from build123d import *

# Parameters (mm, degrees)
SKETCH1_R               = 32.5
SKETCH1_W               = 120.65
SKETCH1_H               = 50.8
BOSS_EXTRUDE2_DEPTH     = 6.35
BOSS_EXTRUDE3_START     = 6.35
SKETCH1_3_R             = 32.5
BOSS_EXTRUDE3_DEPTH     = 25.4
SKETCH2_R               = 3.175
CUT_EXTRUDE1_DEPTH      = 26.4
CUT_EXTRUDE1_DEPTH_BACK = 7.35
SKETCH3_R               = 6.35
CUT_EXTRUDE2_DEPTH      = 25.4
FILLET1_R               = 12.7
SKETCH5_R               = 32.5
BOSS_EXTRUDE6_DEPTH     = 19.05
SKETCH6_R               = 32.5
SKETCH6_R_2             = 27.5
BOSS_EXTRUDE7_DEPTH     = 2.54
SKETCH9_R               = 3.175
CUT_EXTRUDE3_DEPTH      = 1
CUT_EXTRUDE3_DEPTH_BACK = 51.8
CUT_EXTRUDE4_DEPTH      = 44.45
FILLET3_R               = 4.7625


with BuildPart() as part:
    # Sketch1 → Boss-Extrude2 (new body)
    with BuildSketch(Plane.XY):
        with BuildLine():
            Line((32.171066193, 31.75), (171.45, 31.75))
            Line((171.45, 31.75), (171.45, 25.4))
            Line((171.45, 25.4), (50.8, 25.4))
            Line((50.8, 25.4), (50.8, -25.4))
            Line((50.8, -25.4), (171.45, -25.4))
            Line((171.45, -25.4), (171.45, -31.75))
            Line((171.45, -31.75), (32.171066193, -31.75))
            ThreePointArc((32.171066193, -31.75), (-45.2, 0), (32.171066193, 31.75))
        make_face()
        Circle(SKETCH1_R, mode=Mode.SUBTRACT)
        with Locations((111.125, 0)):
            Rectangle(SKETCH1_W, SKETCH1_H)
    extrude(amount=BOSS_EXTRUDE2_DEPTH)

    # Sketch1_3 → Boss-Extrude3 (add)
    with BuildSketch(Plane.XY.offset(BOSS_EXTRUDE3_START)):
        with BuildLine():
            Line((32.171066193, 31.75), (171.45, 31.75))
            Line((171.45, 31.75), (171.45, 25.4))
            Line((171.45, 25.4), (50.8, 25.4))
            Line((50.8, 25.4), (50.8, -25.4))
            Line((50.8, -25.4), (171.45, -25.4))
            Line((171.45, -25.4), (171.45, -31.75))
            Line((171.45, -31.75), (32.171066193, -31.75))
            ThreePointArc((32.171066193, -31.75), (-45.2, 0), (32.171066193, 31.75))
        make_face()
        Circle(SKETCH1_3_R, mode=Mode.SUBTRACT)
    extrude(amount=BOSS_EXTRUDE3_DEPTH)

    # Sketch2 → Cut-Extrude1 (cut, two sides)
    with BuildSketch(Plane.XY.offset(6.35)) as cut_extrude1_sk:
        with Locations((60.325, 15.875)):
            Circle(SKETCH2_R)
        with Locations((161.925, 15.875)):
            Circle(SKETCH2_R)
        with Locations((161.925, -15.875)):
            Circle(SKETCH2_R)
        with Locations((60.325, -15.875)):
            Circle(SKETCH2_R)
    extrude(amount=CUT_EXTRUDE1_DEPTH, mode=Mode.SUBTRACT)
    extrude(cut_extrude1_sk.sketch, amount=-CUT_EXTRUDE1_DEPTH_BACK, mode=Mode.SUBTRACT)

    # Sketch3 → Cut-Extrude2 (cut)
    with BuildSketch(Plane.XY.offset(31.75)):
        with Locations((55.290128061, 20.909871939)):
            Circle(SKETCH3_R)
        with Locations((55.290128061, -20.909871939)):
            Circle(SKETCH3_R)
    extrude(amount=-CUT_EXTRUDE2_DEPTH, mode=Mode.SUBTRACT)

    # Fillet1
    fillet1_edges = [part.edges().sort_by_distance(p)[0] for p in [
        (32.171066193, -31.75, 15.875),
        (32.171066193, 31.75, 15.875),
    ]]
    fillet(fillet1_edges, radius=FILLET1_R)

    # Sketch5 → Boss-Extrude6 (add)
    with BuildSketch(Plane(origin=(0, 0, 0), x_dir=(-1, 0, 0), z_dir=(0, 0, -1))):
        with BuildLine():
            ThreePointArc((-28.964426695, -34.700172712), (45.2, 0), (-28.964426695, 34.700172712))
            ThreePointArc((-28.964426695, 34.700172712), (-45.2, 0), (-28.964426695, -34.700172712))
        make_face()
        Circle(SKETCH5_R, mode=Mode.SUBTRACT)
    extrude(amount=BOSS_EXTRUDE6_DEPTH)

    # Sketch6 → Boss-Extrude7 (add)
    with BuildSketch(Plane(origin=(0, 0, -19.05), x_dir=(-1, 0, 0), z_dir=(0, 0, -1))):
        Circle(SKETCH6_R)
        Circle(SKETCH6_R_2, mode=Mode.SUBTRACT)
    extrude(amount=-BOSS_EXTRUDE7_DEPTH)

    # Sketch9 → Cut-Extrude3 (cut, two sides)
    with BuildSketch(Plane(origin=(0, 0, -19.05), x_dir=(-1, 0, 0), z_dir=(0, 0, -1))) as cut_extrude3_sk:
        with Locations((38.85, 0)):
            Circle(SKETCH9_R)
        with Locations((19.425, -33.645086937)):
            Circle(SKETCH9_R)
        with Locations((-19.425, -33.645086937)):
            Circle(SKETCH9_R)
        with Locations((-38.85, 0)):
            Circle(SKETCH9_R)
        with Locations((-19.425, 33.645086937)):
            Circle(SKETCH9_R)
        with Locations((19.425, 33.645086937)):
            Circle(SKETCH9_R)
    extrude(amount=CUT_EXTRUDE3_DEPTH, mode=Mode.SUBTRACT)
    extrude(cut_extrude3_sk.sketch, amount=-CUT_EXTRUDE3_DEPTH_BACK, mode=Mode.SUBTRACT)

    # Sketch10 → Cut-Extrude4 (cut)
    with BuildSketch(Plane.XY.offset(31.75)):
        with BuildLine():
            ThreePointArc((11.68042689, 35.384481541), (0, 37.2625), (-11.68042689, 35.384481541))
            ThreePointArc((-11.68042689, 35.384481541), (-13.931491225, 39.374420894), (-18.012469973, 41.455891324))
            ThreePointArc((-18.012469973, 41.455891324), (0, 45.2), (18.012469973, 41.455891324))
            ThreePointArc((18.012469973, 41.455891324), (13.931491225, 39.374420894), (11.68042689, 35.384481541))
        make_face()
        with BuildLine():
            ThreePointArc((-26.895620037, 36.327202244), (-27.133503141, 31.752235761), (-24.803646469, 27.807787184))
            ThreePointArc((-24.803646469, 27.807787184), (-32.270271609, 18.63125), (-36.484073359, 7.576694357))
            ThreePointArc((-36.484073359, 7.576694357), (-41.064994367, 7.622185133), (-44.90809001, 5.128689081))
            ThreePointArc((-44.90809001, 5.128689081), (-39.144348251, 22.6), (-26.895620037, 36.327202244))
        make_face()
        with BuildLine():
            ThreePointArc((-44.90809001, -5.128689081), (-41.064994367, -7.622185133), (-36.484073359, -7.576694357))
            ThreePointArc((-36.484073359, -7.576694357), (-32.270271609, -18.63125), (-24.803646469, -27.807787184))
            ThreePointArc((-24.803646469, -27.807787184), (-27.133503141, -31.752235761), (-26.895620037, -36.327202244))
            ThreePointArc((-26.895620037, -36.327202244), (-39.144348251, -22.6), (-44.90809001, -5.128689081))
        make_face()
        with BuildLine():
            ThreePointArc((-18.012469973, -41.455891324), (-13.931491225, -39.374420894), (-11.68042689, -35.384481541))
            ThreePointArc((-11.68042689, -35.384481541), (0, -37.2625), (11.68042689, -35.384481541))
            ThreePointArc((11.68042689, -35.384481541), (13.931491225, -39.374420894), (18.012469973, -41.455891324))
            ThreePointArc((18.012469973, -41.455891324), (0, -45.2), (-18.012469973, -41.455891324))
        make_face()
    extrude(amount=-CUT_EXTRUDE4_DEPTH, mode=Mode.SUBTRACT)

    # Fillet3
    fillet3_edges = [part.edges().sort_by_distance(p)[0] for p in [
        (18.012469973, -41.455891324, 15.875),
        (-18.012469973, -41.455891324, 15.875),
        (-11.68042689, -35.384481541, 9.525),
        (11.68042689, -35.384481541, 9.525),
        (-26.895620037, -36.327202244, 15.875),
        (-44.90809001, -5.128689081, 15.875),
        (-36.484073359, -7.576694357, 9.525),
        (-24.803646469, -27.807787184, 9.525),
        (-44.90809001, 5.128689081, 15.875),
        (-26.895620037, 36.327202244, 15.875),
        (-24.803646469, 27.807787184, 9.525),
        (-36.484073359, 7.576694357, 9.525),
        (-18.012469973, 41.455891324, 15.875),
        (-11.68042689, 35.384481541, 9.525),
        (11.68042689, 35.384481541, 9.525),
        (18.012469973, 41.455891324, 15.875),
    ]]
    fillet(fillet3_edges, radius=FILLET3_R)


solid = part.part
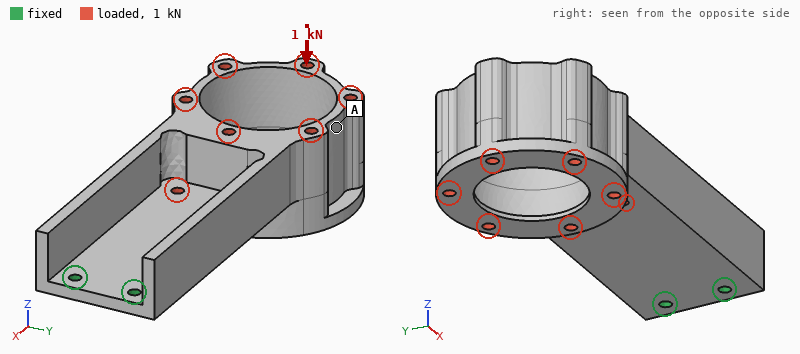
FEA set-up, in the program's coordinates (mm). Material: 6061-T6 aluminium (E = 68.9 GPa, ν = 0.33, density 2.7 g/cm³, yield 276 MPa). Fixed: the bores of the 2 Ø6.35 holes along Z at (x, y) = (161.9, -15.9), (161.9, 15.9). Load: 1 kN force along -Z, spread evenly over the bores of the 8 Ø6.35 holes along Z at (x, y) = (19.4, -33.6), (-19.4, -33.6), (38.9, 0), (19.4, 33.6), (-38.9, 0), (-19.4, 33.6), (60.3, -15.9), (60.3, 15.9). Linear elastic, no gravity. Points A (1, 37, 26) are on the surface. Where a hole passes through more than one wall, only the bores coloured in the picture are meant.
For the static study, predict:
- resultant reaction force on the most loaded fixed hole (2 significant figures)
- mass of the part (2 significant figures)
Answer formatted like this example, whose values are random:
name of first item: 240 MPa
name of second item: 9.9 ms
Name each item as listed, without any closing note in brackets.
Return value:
resultant reaction force on the most loaded fixed hole: 930 N
mass of the part: 580 g
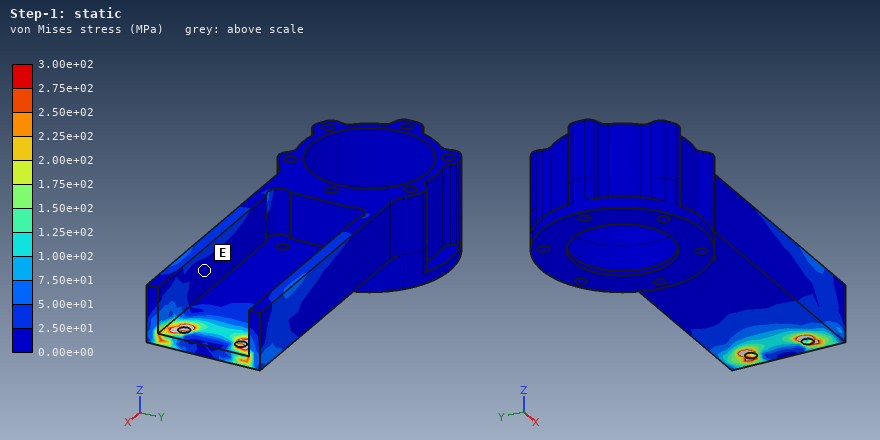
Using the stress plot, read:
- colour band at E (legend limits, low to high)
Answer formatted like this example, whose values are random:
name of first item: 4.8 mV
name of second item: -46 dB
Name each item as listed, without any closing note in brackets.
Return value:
colour band at E: 0.00e+00 to 2.50e+01 MPa
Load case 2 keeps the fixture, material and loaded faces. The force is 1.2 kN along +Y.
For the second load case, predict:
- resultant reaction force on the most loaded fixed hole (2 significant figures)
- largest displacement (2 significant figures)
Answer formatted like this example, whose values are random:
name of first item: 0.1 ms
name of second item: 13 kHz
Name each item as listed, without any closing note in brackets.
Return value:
resultant reaction force on the most loaded fixed hole: 5.3 kN
largest displacement: 0.28 mm
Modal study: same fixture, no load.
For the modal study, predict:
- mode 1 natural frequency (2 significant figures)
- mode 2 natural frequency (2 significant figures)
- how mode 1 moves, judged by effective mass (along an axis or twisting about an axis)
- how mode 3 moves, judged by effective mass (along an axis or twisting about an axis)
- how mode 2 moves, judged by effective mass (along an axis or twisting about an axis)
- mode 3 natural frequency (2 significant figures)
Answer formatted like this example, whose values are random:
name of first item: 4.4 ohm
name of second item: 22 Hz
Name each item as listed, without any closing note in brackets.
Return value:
mode 1 natural frequency: 180 Hz
mode 2 natural frequency: 580 Hz
how mode 1 moves, judged by effective mass: along Z
how mode 3 moves, judged by effective mass: along Y
how mode 2 moves, judged by effective mass: twisting about X
mode 3 natural frequency: 670 Hz
